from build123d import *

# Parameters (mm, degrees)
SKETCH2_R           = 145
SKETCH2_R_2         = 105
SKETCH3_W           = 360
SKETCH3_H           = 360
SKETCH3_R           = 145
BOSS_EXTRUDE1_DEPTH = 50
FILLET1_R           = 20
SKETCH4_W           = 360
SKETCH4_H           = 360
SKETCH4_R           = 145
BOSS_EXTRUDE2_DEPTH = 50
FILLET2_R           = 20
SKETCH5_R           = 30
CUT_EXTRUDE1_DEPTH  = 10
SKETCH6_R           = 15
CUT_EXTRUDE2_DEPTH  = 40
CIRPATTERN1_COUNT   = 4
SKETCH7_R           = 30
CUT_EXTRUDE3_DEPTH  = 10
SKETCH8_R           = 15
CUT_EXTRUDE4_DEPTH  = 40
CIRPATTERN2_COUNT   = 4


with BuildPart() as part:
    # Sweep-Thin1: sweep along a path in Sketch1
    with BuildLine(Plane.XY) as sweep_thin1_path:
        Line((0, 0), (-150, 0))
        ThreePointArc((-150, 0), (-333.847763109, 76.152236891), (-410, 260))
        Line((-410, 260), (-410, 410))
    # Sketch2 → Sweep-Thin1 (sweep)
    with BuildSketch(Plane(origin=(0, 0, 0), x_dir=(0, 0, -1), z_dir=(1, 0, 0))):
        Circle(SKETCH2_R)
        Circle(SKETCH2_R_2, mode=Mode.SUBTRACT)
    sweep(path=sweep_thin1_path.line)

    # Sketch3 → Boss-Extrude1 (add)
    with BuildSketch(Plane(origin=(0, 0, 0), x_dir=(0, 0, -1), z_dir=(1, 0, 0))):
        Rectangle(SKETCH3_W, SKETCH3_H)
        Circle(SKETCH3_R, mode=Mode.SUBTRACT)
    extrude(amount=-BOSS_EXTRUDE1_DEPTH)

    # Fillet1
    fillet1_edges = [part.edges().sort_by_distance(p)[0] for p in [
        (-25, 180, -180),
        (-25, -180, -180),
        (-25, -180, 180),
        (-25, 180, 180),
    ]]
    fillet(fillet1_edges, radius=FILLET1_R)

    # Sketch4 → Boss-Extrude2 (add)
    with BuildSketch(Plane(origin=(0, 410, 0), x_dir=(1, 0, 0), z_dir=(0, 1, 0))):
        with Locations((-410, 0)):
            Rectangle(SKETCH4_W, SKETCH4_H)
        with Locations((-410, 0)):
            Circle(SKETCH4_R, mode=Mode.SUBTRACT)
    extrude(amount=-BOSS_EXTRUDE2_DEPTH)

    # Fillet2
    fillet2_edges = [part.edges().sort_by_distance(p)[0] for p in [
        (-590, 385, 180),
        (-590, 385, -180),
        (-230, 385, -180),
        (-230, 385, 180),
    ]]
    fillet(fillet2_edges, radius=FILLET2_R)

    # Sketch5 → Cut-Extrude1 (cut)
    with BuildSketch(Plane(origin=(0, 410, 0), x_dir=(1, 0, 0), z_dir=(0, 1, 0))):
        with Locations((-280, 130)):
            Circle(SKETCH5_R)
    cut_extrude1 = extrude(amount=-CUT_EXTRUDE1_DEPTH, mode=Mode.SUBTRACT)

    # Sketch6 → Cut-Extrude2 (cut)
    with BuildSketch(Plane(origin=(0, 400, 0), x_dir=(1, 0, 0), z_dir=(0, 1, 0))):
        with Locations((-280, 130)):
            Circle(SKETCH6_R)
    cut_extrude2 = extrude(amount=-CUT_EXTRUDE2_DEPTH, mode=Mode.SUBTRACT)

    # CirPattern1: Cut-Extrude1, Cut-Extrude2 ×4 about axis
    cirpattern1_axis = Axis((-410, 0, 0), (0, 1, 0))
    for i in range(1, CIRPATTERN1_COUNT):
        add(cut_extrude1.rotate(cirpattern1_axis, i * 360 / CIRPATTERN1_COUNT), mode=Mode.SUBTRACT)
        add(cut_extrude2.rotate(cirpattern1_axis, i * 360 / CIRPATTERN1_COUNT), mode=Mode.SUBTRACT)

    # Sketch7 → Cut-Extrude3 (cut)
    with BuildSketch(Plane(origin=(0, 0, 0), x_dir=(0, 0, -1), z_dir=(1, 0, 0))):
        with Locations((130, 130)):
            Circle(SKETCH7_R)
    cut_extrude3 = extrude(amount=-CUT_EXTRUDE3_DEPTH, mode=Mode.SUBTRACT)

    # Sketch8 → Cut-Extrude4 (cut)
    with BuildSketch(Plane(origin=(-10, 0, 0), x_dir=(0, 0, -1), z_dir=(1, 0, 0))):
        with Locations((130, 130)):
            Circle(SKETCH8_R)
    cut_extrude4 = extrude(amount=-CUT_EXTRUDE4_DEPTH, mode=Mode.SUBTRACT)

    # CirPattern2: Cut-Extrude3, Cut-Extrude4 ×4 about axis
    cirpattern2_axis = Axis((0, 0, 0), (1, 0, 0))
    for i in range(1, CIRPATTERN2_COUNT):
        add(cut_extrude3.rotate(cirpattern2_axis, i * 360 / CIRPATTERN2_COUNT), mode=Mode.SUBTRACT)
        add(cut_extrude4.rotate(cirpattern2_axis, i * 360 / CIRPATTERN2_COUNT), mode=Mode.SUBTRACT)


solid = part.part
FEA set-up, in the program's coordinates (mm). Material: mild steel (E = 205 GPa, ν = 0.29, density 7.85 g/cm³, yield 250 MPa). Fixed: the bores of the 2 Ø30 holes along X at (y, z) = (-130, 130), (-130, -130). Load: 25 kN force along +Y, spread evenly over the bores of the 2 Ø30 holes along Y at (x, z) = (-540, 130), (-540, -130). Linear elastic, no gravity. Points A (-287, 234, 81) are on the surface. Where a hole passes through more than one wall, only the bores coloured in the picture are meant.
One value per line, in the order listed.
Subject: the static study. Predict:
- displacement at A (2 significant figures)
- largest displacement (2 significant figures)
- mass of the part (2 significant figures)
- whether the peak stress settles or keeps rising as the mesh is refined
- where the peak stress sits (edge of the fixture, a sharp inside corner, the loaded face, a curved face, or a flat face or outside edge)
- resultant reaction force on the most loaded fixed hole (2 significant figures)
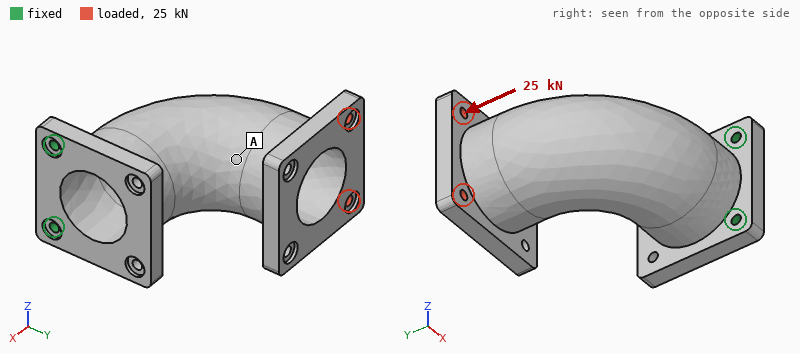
0.74 mm
1.3 mm
220 kg
keeps rising
edge of the fixture
13 kN
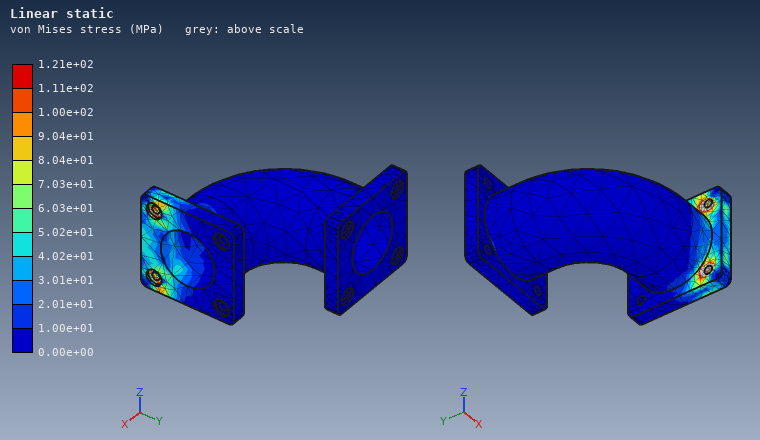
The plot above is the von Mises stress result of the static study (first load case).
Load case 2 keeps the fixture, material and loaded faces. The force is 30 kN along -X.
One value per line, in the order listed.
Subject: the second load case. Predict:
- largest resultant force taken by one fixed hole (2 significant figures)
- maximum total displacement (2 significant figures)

15 kN
1.6 mm
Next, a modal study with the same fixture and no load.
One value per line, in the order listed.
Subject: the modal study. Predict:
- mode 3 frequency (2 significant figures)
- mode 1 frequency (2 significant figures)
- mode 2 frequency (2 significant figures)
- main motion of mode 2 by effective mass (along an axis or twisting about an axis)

550 Hz
69 Hz
220 Hz
along Z
